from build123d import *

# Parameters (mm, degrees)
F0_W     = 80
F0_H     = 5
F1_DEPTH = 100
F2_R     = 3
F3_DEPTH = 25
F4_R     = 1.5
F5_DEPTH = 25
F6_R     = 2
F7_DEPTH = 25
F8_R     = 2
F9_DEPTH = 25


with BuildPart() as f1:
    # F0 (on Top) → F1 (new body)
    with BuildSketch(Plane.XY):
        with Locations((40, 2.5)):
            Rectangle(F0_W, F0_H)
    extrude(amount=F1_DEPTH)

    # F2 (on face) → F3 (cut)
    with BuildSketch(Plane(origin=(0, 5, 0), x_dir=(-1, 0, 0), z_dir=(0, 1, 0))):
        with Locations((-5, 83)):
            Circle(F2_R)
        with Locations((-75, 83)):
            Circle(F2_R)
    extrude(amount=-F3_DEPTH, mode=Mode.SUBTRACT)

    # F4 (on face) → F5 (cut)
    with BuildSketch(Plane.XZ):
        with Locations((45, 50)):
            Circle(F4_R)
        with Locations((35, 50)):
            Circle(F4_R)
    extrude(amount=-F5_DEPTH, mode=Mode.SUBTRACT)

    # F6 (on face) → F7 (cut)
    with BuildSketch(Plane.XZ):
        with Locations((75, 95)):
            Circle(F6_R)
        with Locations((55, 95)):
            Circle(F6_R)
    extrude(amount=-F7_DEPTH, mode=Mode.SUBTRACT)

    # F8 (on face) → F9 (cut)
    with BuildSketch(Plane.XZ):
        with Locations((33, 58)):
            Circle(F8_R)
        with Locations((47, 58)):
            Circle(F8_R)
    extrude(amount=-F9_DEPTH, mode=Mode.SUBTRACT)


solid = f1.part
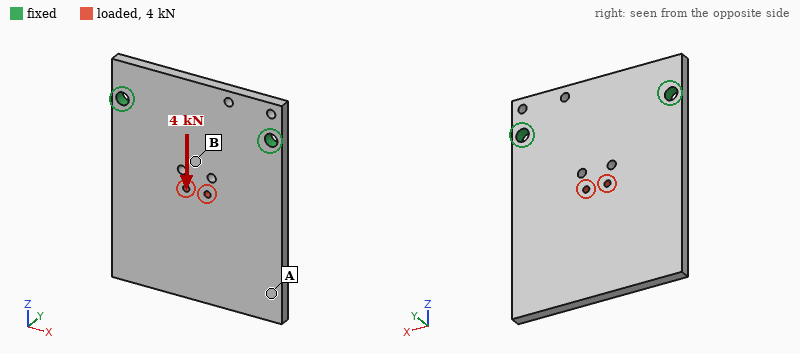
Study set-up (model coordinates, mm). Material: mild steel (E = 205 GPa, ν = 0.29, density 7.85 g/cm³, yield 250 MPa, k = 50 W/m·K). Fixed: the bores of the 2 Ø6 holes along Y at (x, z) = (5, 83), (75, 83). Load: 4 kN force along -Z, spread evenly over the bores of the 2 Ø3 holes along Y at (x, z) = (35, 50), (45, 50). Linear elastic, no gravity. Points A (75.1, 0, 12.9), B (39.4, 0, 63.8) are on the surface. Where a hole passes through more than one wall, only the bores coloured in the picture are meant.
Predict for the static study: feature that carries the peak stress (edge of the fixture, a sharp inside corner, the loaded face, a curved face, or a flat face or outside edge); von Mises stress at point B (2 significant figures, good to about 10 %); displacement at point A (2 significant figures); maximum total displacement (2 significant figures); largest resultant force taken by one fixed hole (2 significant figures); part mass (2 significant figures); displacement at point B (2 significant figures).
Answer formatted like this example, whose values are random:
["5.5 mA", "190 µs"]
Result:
["the loaded face", "14 MPa", "3.0 µm", "5.3 µm", "2.1 kN", "310 g", "3.9 µm"]
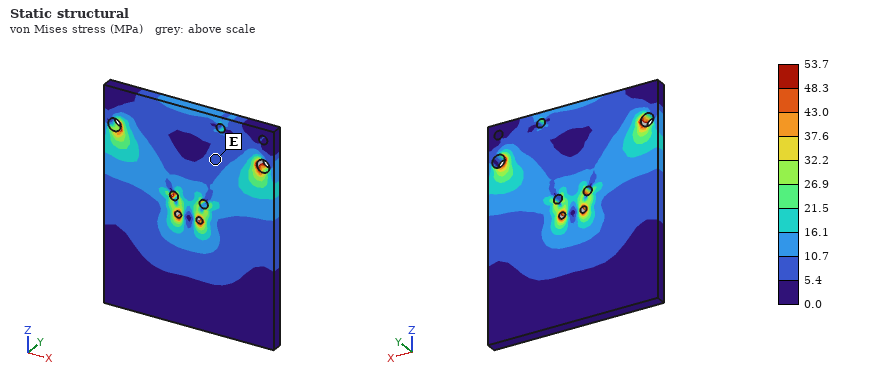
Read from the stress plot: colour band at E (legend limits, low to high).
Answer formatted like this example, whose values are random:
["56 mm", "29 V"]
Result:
["5.4 to 10.7 MPa"]
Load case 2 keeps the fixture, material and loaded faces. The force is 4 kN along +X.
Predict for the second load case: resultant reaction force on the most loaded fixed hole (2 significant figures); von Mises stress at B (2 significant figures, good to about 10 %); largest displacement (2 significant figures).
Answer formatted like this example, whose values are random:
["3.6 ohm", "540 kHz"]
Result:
["2.7 kN", "16 MPa", "9.4 µm"]
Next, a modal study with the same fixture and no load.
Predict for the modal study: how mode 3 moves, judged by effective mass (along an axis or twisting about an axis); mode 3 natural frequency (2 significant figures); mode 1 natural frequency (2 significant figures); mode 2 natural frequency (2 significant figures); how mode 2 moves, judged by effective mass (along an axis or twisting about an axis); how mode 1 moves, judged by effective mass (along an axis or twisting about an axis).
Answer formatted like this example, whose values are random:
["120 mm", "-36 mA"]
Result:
["along Y", "3300 Hz", "530 Hz", "1500 Hz", "twisting about Z", "along Y"]
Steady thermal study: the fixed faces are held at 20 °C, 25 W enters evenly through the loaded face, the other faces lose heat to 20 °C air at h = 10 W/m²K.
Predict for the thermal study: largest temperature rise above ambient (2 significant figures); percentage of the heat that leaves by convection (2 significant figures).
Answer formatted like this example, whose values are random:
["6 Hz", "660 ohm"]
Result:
["70 K", "23 %"]
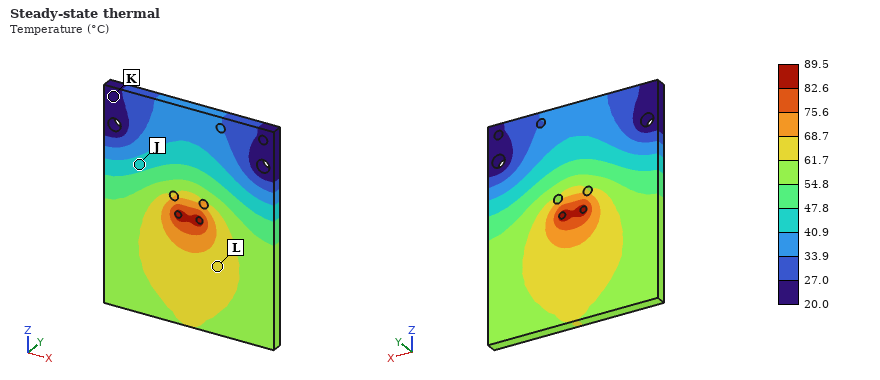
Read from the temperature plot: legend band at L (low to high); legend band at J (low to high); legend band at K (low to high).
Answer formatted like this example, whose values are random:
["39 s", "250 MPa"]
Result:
["61.7 to 68.7 °C", "40.9 to 47.8 °C", "20.0 to 27.0 °C"]
